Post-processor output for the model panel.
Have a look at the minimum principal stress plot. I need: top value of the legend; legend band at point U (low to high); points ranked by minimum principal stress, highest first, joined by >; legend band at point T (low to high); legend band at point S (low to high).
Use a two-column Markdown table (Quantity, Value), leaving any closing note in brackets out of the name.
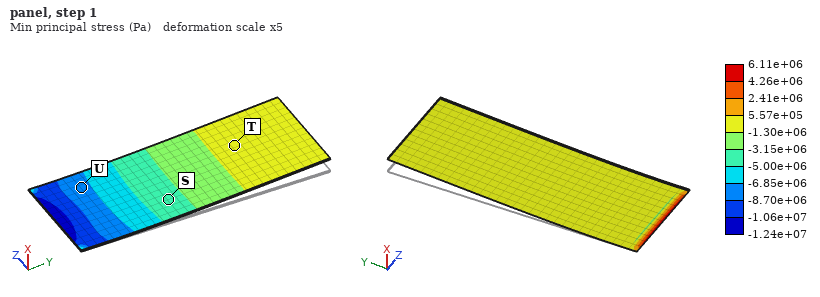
| Quantity | Value |
|---|---|
| top value of the legend | 6.11e+06 Pa |
| legend band at point U | -8.70e+06 to -6.85e+06 Pa |
| points ranked by minimum principal stress, highest first, joined by > | T > S > U |
| legend band at point T | -1.30e+06 to 5.57e+05 Pa |
| legend band at point S | -5.00e+06 to -3.15e+06 Pa |
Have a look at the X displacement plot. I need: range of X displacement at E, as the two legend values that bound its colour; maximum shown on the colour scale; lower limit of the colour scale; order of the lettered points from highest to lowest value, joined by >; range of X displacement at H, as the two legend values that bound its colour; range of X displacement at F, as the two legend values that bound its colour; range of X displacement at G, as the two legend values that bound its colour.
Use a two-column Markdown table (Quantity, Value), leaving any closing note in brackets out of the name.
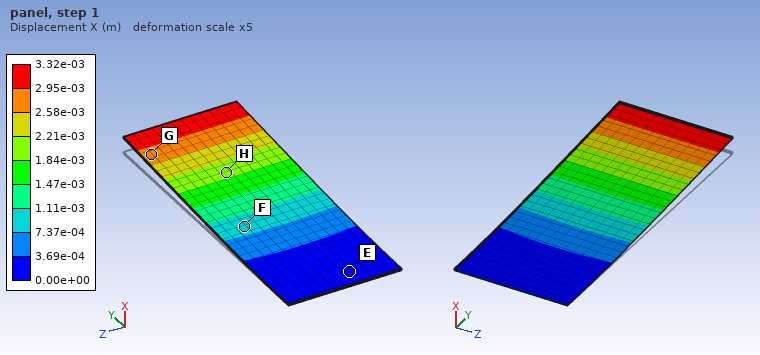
| Quantity | Value |
|---|---|
| range of X displacement at E, as the two legend values that bound its colour | 0.00e+00 to 3.69e-04 m |
| maximum shown on the colour scale | 3.32e-03 m |
| lower limit of the colour scale | 0.00e+00 m |
| order of the lettered points from highest to lowest value, joined by > | G > H > F > E |
| range of X displacement at H, as the two legend values that bound its colour | 1.84e-03 to 2.21e-03 m |
| range of X displacement at F, as the two legend values that bound its colour | 7.37e-04 to 1.11e-03 m |
| range of X displacement at G, as the two legend values that bound its colour | 2.58e-03 to 2.95e-03 m |
